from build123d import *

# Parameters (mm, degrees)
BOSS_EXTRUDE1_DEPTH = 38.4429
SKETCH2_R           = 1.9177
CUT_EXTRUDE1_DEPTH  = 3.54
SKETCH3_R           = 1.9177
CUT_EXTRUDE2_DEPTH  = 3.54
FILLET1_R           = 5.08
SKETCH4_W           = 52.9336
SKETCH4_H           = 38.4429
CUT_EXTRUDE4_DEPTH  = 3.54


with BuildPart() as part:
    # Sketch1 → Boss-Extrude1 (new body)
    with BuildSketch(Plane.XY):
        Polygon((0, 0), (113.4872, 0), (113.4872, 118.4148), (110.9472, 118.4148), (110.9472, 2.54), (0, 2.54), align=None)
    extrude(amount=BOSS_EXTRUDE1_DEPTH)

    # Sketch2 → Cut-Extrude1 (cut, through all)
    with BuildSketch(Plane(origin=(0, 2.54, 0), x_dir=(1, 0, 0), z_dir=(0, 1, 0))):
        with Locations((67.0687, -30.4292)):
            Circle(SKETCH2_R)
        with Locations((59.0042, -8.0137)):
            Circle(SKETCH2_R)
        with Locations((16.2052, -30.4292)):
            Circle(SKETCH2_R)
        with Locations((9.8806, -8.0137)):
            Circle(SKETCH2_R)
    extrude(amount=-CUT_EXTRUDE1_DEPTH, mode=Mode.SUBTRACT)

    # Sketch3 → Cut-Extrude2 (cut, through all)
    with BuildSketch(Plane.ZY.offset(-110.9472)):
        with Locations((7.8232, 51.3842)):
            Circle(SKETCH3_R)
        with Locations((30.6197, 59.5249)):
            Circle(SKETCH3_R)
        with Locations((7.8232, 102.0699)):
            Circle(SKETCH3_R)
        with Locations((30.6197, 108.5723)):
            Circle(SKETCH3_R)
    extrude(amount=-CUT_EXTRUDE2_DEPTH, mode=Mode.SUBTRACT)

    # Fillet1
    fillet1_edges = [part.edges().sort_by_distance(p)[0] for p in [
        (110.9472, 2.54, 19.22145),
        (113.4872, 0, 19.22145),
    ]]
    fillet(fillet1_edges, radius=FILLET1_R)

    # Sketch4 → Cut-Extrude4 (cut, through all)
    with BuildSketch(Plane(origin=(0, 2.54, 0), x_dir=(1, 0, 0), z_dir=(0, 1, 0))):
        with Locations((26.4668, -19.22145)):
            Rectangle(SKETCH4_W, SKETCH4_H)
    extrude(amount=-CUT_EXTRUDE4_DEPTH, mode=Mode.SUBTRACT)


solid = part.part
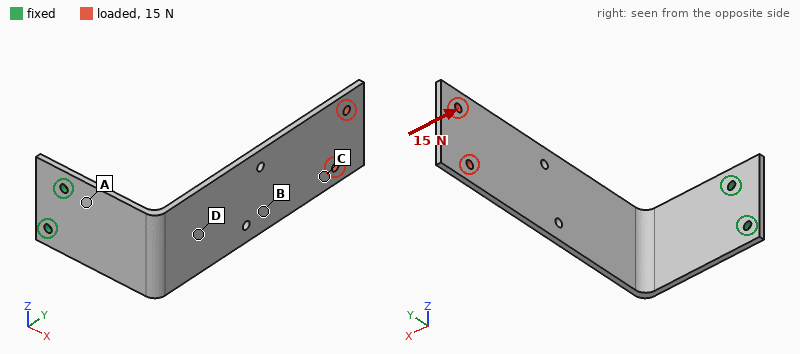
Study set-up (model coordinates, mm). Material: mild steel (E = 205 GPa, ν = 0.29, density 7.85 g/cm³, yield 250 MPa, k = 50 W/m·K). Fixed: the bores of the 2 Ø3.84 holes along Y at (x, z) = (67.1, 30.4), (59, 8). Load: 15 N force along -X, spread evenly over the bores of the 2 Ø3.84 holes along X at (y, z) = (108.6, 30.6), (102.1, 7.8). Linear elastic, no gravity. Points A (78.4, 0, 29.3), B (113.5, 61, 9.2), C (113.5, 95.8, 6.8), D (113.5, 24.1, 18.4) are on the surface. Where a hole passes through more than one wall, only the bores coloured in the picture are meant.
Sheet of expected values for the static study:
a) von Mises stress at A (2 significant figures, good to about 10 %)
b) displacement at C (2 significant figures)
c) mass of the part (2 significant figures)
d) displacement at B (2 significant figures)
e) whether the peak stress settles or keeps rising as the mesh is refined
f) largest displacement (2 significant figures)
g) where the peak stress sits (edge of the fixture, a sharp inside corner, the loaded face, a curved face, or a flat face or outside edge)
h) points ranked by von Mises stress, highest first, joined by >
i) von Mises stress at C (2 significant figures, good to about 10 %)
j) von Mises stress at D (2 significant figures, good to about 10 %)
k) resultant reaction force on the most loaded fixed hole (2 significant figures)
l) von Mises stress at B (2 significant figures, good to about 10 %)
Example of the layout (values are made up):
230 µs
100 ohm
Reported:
37 MPa
1.0 mm
130 g
0.57 mm
keeps rising
1.3 mm
edge of the fixture
A > D > B > C
3.6 MPa
27 MPa
22 N
16 MPa
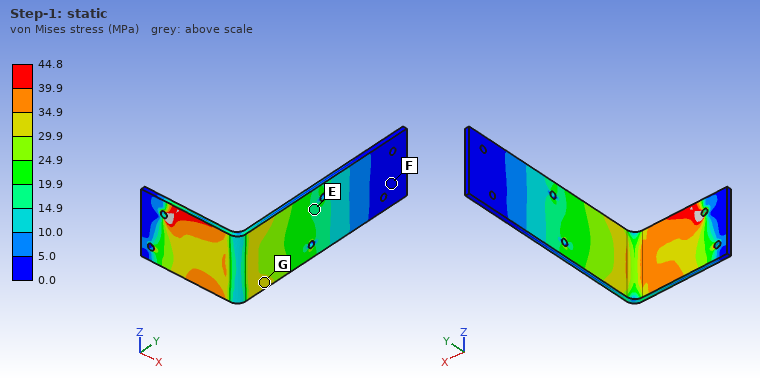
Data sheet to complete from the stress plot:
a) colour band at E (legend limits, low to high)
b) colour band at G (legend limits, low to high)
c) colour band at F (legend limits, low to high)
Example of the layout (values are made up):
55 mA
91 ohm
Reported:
14.9 to 19.9 MPa
29.9 to 34.9 MPa
0.0 to 5.0 MPa
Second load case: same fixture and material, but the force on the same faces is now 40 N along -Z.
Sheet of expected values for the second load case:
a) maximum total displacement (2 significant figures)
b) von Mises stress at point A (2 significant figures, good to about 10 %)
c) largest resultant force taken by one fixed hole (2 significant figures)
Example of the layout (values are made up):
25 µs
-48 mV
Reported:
1.1 mm
77 MPa
150 N
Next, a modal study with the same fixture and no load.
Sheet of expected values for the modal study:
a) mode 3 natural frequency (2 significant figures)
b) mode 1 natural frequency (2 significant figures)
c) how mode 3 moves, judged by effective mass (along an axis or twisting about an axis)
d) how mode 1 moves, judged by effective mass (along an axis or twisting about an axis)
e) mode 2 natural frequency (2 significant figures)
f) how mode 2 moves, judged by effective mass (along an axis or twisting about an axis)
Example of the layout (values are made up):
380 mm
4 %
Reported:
390 Hz
97 Hz
along Y
along X
170 Hz
along Z
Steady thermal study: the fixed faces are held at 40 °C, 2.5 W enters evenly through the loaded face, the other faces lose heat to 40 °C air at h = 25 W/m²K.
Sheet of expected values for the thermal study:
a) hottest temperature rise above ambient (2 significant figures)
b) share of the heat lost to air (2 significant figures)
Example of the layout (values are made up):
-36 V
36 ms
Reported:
22 K
93 %
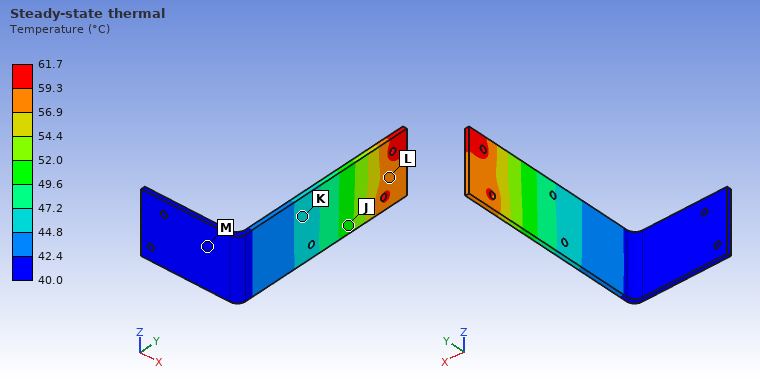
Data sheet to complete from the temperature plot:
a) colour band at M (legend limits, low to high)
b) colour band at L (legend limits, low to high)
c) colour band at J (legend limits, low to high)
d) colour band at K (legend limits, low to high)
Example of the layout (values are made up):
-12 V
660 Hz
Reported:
40.0 to 42.4 °C
56.9 to 59.3 °C
49.6 to 52.0 °C
44.8 to 47.2 °C
